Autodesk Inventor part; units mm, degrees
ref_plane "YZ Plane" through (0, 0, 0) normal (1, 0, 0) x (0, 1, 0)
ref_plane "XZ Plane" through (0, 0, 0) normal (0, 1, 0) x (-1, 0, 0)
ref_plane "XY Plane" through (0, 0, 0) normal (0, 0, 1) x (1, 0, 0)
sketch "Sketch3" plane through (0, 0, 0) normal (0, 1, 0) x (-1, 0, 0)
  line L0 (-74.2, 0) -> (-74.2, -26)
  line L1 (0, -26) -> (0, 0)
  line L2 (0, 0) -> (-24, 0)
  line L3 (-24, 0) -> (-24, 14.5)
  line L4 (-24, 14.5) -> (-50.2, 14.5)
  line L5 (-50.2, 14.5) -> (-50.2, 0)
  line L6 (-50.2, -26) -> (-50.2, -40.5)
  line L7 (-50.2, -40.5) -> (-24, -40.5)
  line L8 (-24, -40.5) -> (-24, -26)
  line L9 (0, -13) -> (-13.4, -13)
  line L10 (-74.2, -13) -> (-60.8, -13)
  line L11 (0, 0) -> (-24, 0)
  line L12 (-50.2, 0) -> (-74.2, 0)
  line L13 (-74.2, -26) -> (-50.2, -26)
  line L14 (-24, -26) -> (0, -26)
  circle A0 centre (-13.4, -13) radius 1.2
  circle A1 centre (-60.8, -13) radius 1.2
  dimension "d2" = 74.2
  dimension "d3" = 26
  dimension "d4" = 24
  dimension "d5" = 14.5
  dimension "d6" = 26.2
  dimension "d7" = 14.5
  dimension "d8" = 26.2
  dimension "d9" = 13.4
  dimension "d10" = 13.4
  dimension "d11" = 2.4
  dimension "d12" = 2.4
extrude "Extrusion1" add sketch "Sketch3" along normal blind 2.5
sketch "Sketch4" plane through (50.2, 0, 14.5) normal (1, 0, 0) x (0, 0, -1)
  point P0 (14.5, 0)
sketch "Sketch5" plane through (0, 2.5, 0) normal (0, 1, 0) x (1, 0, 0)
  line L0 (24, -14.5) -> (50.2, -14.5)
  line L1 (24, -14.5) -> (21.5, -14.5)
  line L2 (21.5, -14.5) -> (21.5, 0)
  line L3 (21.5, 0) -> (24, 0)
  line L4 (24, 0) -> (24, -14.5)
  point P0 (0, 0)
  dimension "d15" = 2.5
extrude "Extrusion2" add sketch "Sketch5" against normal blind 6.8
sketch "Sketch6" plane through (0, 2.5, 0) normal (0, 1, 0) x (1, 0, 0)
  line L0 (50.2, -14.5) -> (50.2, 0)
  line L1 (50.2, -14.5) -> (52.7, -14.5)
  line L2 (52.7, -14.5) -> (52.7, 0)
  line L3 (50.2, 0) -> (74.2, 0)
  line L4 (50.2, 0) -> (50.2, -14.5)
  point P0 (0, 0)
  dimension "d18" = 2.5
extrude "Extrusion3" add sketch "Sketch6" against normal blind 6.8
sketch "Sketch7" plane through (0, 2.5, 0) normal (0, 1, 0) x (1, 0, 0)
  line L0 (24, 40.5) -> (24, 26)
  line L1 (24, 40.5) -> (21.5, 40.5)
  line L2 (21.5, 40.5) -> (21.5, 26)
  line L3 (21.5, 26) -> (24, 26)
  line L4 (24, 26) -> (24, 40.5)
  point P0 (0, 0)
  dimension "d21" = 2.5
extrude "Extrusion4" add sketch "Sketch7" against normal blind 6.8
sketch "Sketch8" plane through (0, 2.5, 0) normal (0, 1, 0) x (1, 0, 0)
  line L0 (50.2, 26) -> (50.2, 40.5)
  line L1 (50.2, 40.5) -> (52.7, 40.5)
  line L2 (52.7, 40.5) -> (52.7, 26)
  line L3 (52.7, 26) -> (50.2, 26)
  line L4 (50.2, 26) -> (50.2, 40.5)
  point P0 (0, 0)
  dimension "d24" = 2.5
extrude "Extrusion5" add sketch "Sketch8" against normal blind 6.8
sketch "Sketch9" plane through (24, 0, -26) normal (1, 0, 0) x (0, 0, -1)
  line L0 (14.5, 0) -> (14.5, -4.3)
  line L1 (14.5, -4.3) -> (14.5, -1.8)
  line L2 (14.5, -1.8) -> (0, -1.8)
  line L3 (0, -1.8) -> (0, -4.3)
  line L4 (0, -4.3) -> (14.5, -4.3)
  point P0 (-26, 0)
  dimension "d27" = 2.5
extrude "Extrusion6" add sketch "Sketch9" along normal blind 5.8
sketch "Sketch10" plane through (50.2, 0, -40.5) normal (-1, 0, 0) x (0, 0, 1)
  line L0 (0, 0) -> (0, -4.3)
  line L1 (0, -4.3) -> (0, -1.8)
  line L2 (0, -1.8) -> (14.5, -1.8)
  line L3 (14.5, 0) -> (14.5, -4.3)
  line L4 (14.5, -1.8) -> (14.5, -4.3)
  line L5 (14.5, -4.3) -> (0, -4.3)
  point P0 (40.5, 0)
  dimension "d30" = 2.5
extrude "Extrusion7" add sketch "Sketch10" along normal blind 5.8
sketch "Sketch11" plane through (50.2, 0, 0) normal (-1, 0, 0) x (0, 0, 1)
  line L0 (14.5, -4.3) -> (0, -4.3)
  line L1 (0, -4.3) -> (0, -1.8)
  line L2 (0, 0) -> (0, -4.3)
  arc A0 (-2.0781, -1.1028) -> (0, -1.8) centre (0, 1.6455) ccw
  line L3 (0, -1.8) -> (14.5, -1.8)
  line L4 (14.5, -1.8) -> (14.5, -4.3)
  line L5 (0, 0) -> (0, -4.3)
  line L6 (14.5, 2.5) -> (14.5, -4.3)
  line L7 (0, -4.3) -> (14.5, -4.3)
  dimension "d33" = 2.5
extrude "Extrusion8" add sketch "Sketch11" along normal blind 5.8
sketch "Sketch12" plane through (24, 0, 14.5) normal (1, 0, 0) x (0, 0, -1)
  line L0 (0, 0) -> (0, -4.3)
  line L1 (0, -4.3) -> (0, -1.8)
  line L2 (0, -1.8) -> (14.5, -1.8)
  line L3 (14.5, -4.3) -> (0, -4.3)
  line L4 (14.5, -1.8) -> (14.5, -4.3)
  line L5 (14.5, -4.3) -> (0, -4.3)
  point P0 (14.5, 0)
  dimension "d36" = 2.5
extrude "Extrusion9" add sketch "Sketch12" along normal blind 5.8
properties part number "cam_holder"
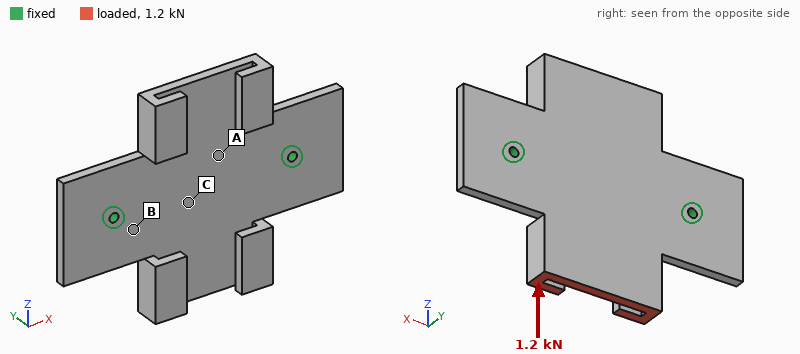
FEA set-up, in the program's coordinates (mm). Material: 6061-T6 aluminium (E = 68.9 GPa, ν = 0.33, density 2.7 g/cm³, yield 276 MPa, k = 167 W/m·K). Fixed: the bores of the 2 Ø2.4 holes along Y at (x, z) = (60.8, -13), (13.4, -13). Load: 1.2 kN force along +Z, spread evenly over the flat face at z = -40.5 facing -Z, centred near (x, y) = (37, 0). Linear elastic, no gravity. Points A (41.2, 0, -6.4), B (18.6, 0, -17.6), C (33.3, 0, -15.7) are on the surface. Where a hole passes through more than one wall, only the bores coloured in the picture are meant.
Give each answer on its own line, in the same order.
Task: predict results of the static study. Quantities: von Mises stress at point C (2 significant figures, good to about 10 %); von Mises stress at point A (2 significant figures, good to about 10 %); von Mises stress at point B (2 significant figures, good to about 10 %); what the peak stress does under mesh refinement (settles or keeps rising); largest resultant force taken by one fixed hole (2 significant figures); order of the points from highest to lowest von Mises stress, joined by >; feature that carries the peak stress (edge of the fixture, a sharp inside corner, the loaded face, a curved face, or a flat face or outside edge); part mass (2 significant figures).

29 MPa
14 MPa
53 MPa
keeps rising
610 N
B > C > A
edge of the fixture
23 g
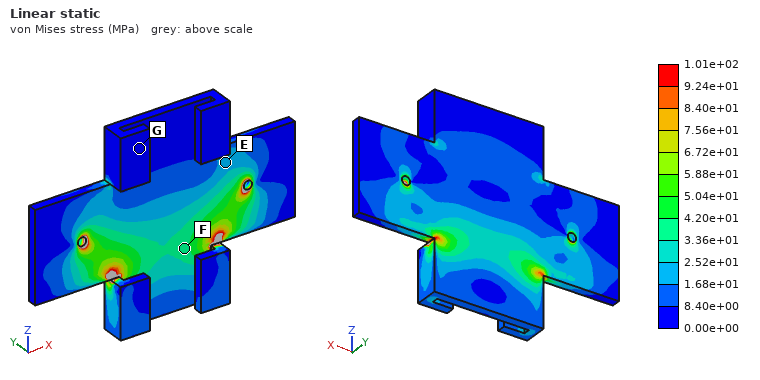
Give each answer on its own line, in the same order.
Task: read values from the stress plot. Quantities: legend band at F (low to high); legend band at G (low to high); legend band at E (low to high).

3.36e+01 to 4.20e+01 MPa
0.00e+00 to 8.40e+00 MPa
1.68e+01 to 2.52e+01 MPa
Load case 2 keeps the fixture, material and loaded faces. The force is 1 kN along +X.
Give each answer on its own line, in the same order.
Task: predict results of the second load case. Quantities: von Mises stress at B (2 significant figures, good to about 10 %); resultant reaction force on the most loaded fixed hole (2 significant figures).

31 MPa
770 N
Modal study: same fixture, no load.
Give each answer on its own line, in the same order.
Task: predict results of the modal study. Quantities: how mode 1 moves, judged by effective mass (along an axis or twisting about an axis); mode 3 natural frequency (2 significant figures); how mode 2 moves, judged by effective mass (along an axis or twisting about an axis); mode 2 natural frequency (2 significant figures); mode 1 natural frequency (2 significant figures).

twisting about X
4400 Hz
along Y
2200 Hz
1600 Hz
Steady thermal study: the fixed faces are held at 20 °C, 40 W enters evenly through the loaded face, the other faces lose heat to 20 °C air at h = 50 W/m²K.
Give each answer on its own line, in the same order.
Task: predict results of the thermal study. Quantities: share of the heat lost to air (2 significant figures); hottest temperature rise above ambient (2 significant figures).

24 %
75 K
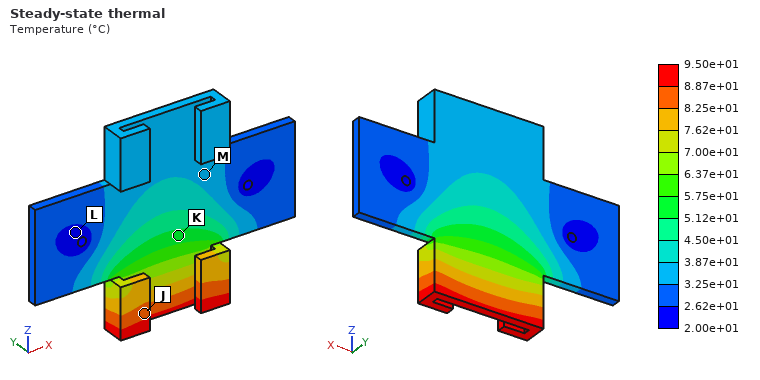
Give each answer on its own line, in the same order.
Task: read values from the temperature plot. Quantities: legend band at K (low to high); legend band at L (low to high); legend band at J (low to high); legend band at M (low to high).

5.12e+01 to 5.75e+01 °C
2.00e+01 to 2.62e+01 °C
8.25e+01 to 8.87e+01 °C
3.25e+01 to 3.87e+01 °C
